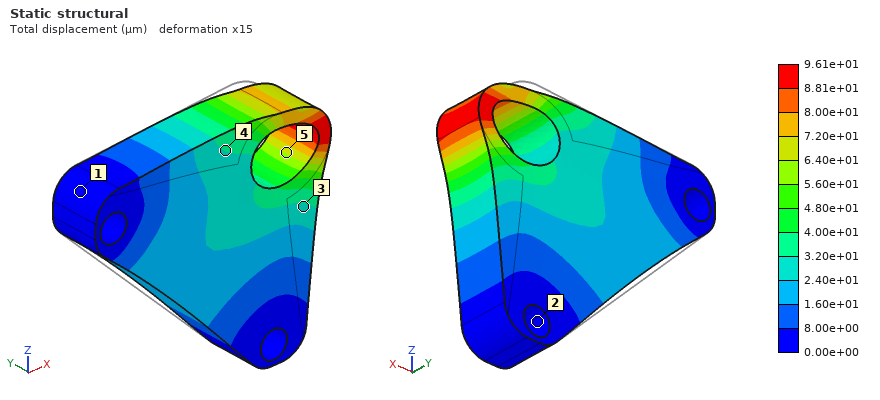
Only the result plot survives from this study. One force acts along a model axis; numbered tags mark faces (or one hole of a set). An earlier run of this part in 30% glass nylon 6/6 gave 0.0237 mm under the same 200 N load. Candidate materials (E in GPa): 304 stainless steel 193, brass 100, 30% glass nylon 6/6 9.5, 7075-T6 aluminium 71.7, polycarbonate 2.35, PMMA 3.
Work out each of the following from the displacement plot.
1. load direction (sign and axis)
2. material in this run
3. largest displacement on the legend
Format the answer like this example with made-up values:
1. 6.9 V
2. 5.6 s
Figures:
1. +X
2. polycarbonate
3. 9.61e+01 µm
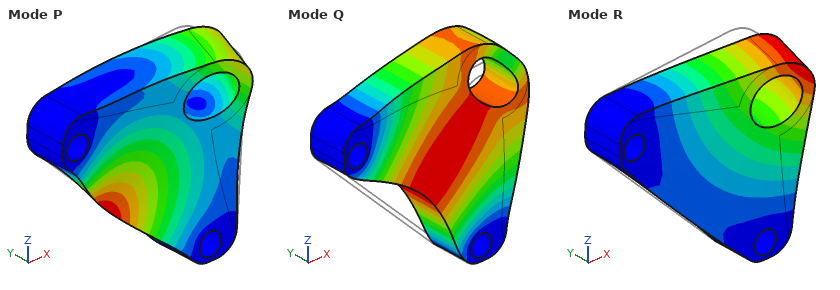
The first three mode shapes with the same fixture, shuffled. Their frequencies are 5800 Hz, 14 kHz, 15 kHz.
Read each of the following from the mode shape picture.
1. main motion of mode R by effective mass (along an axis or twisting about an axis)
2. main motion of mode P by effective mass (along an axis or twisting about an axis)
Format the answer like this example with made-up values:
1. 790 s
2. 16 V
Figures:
1. along Y
2. along Y
